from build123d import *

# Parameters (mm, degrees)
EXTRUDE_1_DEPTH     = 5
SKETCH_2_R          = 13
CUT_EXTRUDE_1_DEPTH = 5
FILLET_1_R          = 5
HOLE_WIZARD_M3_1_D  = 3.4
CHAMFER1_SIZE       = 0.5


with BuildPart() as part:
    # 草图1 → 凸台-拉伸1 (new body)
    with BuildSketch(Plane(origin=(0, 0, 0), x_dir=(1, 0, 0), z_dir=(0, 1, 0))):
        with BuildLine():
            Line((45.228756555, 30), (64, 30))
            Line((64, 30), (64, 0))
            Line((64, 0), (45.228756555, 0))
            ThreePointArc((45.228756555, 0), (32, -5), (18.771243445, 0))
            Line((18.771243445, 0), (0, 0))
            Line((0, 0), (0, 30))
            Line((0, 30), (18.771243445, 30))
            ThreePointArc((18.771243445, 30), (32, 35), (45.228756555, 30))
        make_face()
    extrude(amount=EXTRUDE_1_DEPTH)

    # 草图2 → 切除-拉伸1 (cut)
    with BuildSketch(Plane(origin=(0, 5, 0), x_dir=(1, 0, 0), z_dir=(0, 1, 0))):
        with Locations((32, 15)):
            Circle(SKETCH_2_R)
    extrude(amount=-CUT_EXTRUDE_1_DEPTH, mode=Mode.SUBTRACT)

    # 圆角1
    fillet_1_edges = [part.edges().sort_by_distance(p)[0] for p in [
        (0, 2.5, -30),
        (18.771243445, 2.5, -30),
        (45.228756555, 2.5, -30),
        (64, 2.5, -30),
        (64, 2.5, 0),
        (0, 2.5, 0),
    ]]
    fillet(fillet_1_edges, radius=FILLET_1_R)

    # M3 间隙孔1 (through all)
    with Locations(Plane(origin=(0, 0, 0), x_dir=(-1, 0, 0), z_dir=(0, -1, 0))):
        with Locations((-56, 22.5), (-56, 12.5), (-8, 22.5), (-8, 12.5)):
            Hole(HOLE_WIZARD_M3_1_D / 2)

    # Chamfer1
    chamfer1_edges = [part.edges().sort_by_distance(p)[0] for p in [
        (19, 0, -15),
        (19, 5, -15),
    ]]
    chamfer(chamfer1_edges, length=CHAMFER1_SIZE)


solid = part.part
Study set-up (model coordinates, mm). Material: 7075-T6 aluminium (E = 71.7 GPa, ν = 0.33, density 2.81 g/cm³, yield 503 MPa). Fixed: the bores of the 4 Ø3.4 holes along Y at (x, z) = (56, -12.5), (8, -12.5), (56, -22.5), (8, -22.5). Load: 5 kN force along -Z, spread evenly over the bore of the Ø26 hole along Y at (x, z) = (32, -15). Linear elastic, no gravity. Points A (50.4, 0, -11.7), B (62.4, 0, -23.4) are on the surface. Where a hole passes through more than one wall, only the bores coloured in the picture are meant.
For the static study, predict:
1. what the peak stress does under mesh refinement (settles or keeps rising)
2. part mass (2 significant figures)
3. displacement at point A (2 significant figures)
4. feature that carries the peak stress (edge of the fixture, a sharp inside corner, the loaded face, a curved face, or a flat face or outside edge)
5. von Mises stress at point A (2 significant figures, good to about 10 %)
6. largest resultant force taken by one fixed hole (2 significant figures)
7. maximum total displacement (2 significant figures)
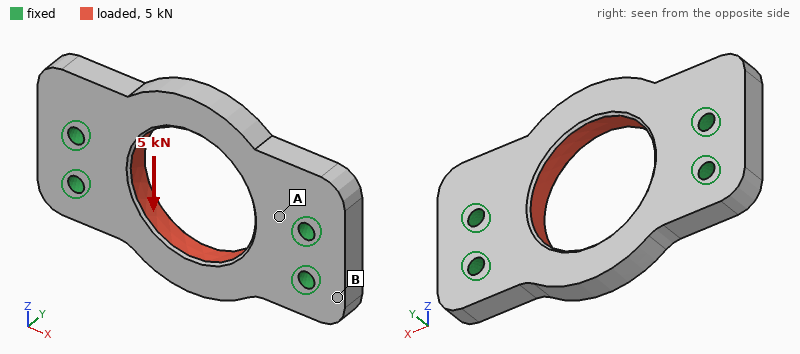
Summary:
keeps rising
21 g
5.3 µm
edge of the fixture
36 MPa
1.5 kN
20 µm
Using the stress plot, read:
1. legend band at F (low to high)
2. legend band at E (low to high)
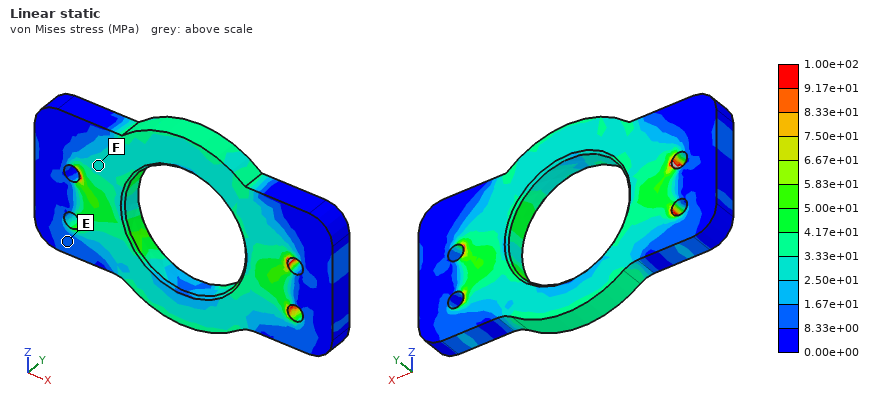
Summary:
2.50e+01 to 3.33e+01 MPa
8.33e+00 to 1.67e+01 MPa
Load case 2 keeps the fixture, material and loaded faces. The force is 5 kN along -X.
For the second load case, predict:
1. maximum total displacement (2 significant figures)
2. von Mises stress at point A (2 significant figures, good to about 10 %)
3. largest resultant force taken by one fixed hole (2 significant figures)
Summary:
12 µm
27 MPa
1.6 kN
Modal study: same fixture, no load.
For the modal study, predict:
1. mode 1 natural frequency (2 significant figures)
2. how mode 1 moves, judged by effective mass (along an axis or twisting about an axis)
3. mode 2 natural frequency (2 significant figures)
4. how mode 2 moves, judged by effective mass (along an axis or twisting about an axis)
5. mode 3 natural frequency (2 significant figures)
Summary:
8700 Hz
along Y
11 kHz
along Y
20 kHz
